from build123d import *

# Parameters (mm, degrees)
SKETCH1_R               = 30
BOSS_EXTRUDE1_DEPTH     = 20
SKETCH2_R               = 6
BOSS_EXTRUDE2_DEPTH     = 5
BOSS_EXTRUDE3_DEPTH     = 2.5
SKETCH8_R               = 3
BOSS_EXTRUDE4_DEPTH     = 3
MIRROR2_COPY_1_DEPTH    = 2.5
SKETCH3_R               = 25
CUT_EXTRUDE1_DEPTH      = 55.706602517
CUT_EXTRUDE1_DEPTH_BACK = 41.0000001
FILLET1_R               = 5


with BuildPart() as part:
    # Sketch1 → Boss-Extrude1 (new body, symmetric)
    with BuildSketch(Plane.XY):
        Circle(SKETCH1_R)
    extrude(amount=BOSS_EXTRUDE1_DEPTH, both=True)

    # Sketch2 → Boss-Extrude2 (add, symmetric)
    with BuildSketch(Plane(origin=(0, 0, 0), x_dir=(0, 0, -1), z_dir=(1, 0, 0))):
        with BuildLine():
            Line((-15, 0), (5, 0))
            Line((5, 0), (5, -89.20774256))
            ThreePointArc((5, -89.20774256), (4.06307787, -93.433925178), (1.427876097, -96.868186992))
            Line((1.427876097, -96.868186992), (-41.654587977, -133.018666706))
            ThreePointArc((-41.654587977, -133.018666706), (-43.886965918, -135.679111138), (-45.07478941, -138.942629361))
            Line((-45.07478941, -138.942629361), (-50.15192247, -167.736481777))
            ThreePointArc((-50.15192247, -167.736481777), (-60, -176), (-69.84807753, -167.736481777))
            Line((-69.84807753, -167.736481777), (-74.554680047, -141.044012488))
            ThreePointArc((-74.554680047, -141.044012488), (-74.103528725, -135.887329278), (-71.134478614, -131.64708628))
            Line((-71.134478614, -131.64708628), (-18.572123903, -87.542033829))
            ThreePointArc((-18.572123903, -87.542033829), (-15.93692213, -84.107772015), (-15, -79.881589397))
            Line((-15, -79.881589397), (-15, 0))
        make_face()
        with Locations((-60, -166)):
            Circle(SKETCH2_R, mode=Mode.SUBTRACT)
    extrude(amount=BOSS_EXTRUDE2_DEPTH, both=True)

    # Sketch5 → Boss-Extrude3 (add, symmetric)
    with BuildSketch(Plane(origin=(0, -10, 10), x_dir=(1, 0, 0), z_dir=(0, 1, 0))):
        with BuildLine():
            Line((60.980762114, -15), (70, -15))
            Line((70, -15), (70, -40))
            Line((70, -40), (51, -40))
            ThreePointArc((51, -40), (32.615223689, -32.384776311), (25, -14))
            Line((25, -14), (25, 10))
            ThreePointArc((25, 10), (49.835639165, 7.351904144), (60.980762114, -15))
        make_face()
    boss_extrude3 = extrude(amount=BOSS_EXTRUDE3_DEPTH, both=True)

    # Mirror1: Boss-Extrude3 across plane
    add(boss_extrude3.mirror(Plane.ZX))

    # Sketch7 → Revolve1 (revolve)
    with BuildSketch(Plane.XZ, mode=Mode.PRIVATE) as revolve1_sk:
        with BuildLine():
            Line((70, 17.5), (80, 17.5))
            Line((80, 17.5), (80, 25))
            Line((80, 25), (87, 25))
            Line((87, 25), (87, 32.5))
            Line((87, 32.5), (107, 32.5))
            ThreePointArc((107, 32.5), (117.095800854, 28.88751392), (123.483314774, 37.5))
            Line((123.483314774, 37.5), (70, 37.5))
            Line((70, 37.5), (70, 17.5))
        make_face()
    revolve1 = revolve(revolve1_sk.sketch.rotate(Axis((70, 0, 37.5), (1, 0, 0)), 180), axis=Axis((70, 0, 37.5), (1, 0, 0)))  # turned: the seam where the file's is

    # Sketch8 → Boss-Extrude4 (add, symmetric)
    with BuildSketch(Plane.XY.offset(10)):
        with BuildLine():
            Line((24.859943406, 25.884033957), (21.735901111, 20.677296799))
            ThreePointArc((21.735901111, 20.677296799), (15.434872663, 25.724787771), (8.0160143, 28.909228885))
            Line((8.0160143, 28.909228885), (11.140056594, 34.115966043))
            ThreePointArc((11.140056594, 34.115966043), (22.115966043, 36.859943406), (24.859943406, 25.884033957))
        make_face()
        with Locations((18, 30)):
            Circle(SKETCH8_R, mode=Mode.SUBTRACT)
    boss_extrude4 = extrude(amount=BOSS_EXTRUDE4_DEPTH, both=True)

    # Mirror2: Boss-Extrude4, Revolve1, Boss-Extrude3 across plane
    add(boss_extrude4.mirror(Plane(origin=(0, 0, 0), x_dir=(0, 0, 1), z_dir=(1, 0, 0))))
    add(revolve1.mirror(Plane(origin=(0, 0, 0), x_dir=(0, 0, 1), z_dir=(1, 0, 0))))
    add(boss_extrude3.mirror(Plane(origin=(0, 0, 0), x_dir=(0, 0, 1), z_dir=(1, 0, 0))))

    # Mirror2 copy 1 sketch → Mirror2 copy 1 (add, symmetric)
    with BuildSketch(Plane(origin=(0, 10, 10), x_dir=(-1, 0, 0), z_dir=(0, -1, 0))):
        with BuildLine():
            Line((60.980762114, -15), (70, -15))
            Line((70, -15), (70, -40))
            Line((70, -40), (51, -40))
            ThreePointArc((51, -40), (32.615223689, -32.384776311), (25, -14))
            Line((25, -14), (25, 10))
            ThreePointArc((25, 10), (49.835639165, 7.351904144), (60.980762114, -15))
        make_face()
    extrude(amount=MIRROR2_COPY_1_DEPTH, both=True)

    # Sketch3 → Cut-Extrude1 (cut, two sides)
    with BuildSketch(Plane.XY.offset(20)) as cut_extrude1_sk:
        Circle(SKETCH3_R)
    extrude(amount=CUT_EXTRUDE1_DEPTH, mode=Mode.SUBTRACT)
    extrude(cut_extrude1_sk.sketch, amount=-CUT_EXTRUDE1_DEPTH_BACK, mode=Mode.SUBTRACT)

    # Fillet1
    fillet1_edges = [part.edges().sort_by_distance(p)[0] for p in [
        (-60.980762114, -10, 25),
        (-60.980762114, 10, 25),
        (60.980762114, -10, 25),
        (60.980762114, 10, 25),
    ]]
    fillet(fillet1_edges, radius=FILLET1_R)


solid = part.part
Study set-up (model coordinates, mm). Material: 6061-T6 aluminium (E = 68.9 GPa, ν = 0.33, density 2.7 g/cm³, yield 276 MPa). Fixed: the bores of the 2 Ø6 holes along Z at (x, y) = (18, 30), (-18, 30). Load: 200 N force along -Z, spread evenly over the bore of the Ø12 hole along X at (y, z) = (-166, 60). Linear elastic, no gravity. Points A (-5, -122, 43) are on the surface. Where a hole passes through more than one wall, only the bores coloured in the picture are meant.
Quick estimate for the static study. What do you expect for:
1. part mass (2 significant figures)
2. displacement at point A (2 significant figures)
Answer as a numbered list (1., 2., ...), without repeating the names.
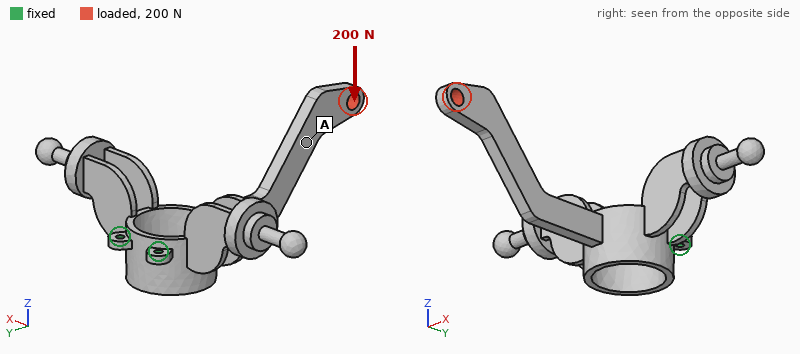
1. 400 g
2. 1.8 mm
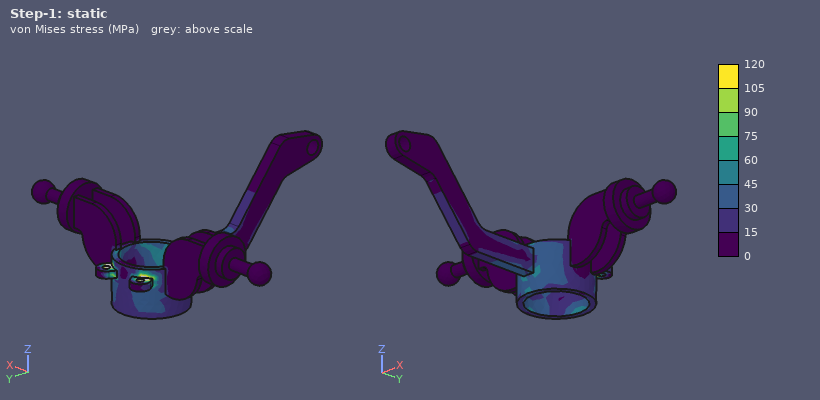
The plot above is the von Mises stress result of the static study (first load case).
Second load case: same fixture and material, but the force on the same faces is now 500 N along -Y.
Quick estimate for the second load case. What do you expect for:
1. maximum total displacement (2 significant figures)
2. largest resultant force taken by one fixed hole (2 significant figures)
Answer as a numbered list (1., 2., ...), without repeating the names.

1. 2.3 mm
2. 250 N
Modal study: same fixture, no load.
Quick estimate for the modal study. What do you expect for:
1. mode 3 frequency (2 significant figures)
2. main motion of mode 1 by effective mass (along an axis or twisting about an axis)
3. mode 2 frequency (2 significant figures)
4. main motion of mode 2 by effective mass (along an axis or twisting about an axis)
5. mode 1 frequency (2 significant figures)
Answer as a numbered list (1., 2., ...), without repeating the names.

1. 430 Hz
2. along Z
3. 260 Hz
4. along X
5. 210 Hz
